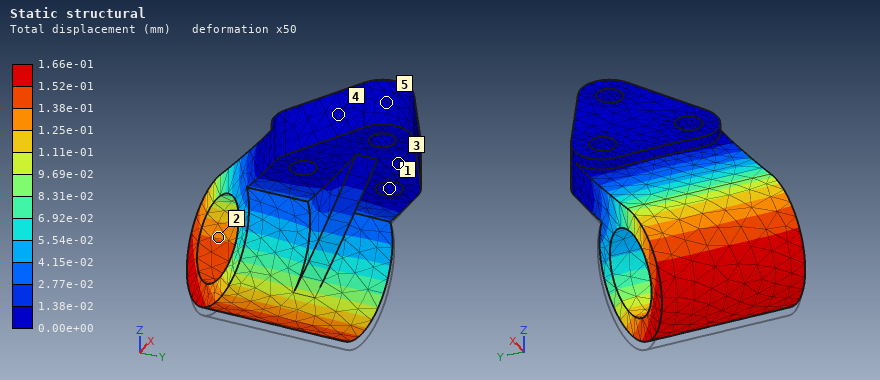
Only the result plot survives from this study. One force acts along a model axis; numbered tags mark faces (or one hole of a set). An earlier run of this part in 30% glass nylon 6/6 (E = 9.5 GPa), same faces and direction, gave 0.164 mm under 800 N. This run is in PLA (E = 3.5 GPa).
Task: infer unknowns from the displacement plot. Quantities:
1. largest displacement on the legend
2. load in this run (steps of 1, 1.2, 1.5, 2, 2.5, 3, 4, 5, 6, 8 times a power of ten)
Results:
1.66e-01 mm
300 N
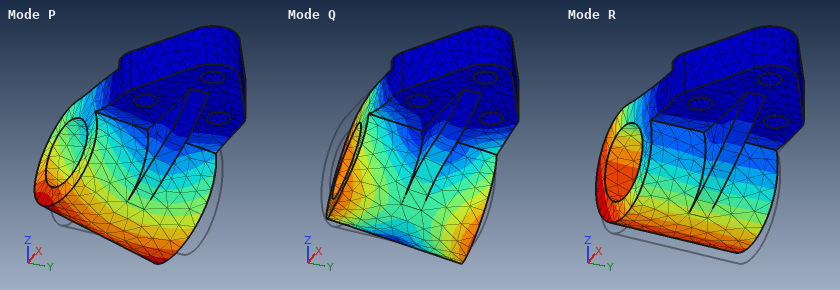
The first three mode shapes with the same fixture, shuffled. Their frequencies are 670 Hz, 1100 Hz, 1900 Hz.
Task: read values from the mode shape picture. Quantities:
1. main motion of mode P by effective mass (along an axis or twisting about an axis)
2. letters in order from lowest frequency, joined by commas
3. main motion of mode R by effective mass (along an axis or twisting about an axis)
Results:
along Y
R, P, Q
along Z
